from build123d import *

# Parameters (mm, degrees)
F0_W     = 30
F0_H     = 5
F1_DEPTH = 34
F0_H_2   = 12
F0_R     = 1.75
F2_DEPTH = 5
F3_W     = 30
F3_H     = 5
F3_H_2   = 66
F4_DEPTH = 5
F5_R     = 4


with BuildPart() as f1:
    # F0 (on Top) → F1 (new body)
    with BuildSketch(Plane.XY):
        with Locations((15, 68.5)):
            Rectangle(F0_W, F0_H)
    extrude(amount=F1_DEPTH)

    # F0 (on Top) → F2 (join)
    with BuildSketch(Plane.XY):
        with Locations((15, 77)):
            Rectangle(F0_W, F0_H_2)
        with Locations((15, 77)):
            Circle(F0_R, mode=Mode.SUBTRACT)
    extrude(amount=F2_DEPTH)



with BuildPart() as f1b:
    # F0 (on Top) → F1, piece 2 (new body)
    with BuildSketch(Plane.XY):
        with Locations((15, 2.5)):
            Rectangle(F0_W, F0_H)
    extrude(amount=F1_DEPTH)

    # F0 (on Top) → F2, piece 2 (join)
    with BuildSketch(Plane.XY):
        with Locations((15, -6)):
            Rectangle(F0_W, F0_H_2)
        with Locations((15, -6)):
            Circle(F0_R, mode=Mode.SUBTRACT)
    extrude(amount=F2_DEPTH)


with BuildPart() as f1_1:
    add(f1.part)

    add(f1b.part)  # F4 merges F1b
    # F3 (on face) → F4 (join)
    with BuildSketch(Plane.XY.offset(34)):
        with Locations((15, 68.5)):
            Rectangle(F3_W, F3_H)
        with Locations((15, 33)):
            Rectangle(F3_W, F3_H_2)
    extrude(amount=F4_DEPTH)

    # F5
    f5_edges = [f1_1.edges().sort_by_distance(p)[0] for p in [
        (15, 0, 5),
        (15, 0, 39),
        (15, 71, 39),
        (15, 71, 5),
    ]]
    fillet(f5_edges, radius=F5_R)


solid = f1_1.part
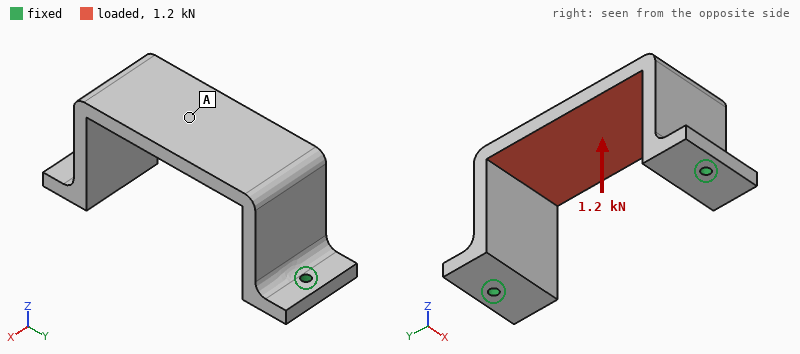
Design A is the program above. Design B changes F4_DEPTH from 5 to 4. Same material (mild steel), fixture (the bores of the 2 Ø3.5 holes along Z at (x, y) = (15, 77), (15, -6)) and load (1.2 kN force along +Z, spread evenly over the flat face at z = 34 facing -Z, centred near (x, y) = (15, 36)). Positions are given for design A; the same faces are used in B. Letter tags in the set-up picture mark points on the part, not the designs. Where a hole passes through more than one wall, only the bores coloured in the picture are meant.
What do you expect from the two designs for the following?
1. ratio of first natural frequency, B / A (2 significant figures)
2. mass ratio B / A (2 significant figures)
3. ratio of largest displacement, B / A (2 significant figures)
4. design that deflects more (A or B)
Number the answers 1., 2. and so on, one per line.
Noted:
1. 1.1
2. 0.91
3. 1.5
4. B
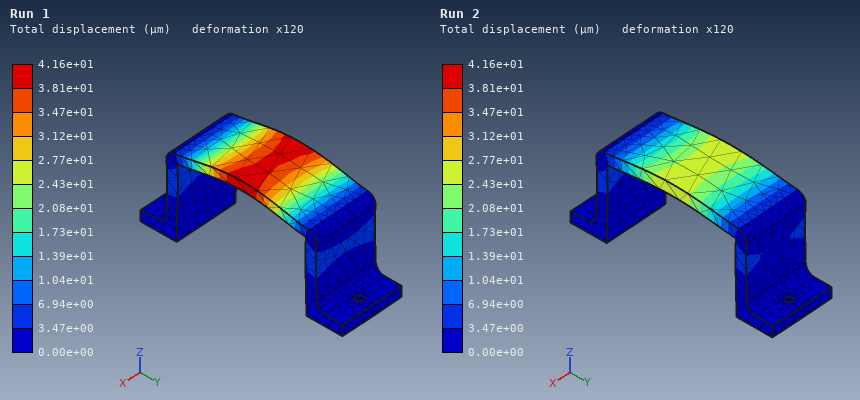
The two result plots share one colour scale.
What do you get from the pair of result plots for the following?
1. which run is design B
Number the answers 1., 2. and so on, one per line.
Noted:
1. Run 1
